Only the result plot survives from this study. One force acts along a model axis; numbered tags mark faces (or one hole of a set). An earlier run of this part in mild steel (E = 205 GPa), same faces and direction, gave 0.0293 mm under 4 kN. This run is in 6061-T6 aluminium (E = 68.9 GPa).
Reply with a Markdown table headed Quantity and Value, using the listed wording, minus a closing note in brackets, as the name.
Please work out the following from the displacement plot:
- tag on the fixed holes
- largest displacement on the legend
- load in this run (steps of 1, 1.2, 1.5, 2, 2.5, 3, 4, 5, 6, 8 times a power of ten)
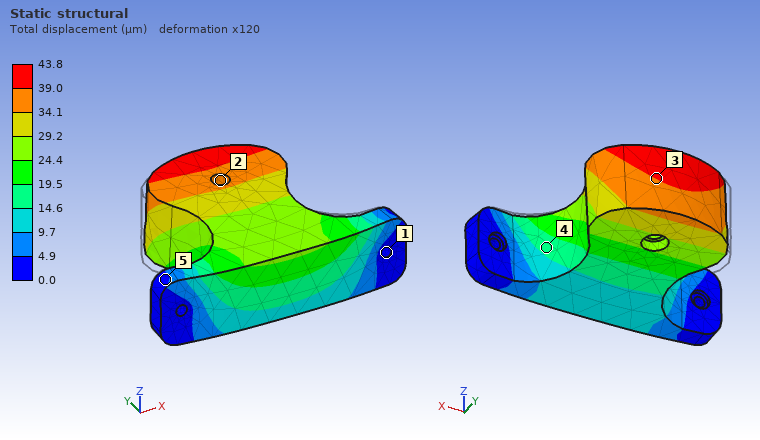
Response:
| Quantity | Value |
|---|---|
| tag on the fixed holes | 1 |
| largest displacement on the legend | 43.8 µm |
| load in this run | 2 kN |
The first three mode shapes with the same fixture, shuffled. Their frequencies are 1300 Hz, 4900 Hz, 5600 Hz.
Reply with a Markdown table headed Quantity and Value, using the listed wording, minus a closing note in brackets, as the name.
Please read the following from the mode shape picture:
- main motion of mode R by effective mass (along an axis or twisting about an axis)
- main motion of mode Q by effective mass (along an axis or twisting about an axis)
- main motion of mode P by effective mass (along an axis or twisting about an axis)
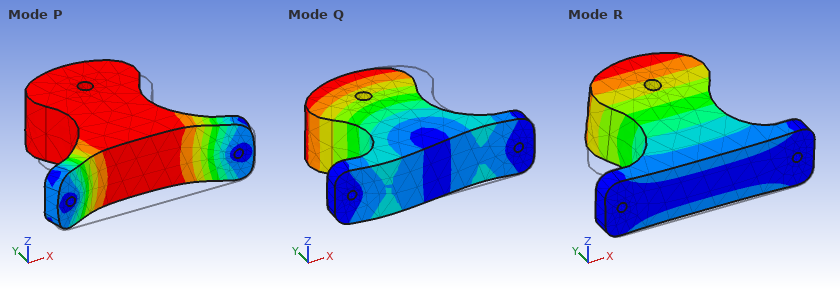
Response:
| Quantity | Value |
|---|---|
| main motion of mode R by effective mass | along Z |
| main motion of mode Q by effective mass | along X |
| main motion of mode P by effective mass | along Y |
